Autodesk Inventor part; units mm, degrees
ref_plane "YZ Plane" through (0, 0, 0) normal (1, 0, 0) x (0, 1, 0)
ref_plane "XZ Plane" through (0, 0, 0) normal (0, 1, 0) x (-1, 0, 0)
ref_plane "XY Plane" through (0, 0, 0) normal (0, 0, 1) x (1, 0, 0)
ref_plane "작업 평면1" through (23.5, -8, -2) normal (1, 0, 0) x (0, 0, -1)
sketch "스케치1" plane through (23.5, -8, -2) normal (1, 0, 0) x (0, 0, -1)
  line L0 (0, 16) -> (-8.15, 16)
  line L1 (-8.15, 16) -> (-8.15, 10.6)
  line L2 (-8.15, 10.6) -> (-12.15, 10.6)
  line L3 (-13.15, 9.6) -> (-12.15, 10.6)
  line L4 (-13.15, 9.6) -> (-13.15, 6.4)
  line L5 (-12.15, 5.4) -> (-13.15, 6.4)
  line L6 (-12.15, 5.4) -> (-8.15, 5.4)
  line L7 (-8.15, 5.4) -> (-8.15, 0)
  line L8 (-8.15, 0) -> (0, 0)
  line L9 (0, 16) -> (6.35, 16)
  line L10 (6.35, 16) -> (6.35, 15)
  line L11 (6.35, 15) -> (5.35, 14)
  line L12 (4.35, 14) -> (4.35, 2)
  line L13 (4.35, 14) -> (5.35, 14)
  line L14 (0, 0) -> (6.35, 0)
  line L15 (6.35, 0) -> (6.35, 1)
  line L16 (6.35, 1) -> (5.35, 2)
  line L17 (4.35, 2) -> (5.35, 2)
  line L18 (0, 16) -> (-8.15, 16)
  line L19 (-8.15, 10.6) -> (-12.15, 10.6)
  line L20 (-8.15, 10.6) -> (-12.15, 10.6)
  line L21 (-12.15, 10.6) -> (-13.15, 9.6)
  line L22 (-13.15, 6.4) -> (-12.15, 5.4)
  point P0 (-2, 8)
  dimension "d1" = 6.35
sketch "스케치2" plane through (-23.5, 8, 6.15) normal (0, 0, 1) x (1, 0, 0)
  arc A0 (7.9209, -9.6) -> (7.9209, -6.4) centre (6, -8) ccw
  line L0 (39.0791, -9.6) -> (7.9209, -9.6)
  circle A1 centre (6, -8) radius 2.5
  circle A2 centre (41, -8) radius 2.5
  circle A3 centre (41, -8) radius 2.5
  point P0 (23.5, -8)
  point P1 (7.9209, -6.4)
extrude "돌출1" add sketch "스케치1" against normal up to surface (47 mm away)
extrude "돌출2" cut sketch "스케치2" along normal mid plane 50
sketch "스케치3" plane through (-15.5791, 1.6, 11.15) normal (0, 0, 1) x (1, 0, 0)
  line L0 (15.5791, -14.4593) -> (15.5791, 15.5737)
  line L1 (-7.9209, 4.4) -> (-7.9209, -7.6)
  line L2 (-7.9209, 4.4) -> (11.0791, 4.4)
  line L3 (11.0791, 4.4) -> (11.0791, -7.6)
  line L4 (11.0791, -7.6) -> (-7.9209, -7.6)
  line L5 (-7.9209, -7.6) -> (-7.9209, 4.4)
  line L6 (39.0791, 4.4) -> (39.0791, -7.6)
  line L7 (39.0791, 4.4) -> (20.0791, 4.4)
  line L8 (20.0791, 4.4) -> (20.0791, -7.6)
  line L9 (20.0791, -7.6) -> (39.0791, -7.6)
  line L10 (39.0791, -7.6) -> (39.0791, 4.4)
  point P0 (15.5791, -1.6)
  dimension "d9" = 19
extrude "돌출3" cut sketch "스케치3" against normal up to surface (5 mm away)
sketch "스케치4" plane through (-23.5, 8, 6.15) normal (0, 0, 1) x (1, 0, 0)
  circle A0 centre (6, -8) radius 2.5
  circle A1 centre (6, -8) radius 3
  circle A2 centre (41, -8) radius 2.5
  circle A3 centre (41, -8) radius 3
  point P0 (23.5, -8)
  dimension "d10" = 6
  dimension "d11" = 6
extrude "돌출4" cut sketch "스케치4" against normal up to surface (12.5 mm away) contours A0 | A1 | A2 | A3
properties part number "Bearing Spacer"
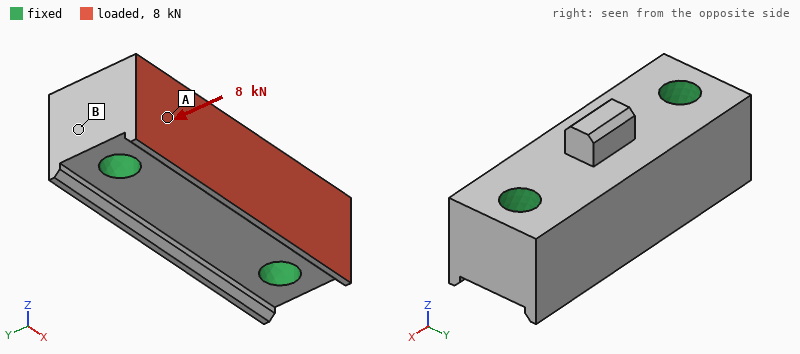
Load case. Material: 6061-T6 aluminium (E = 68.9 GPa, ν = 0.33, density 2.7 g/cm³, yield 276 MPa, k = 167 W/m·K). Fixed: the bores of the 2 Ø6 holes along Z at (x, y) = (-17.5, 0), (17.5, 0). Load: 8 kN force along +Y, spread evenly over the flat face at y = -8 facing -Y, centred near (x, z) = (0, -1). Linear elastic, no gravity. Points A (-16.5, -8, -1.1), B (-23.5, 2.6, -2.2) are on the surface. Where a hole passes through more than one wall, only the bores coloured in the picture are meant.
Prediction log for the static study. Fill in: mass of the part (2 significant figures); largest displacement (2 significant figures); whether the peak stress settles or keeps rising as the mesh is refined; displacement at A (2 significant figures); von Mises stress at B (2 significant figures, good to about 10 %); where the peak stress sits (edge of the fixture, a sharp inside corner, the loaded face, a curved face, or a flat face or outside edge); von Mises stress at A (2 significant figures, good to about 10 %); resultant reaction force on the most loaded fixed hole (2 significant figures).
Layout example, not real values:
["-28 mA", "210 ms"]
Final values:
["25 g", "15 µm", "keeps rising", "2.3 µm", "8.2 MPa", "edge of the fixture", "27 MPa", "4.0 kN"]
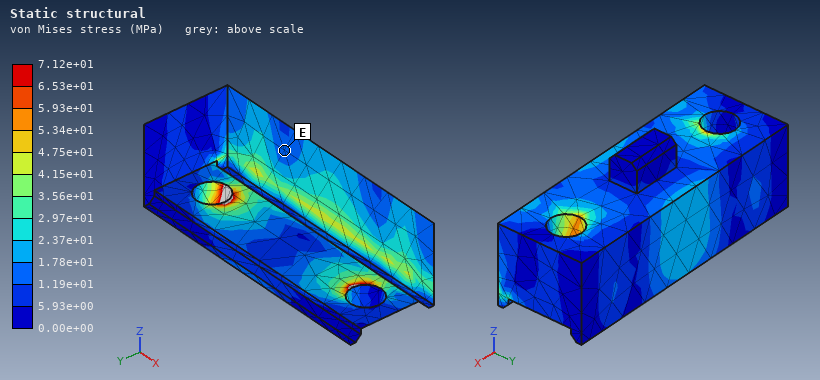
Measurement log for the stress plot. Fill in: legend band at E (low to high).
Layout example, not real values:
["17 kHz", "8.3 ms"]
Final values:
["1.19e+01 to 1.78e+01 MPa"]
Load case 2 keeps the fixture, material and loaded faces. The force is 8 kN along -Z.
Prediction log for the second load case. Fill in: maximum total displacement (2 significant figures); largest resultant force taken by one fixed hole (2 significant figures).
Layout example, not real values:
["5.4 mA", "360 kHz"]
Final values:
["29 µm", "4.0 kN"]
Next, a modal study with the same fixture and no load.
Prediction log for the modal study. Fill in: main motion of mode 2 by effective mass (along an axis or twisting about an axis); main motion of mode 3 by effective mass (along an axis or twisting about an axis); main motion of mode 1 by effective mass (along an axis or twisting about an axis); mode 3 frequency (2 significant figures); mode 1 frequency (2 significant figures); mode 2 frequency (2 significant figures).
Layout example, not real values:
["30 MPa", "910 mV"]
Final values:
["along Z", "twisting about X", "along Y", "38 kHz", "33 kHz", "34 kHz"]
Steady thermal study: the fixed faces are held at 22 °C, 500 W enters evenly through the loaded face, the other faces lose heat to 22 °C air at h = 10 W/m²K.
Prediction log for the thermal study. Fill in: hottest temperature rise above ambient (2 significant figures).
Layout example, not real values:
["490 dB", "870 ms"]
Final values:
["81 K"]
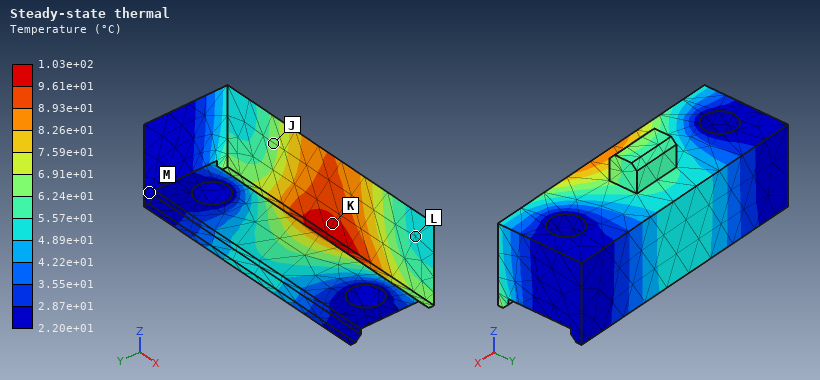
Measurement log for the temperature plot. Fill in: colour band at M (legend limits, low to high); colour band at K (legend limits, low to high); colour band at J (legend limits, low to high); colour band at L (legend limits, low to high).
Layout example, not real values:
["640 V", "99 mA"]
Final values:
["2.20e+01 to 2.87e+01 °C", "9.61e+01 to 1.03e+02 °C", "6.24e+01 to 6.91e+01 °C", "4.89e+01 to 5.57e+01 °C"]
